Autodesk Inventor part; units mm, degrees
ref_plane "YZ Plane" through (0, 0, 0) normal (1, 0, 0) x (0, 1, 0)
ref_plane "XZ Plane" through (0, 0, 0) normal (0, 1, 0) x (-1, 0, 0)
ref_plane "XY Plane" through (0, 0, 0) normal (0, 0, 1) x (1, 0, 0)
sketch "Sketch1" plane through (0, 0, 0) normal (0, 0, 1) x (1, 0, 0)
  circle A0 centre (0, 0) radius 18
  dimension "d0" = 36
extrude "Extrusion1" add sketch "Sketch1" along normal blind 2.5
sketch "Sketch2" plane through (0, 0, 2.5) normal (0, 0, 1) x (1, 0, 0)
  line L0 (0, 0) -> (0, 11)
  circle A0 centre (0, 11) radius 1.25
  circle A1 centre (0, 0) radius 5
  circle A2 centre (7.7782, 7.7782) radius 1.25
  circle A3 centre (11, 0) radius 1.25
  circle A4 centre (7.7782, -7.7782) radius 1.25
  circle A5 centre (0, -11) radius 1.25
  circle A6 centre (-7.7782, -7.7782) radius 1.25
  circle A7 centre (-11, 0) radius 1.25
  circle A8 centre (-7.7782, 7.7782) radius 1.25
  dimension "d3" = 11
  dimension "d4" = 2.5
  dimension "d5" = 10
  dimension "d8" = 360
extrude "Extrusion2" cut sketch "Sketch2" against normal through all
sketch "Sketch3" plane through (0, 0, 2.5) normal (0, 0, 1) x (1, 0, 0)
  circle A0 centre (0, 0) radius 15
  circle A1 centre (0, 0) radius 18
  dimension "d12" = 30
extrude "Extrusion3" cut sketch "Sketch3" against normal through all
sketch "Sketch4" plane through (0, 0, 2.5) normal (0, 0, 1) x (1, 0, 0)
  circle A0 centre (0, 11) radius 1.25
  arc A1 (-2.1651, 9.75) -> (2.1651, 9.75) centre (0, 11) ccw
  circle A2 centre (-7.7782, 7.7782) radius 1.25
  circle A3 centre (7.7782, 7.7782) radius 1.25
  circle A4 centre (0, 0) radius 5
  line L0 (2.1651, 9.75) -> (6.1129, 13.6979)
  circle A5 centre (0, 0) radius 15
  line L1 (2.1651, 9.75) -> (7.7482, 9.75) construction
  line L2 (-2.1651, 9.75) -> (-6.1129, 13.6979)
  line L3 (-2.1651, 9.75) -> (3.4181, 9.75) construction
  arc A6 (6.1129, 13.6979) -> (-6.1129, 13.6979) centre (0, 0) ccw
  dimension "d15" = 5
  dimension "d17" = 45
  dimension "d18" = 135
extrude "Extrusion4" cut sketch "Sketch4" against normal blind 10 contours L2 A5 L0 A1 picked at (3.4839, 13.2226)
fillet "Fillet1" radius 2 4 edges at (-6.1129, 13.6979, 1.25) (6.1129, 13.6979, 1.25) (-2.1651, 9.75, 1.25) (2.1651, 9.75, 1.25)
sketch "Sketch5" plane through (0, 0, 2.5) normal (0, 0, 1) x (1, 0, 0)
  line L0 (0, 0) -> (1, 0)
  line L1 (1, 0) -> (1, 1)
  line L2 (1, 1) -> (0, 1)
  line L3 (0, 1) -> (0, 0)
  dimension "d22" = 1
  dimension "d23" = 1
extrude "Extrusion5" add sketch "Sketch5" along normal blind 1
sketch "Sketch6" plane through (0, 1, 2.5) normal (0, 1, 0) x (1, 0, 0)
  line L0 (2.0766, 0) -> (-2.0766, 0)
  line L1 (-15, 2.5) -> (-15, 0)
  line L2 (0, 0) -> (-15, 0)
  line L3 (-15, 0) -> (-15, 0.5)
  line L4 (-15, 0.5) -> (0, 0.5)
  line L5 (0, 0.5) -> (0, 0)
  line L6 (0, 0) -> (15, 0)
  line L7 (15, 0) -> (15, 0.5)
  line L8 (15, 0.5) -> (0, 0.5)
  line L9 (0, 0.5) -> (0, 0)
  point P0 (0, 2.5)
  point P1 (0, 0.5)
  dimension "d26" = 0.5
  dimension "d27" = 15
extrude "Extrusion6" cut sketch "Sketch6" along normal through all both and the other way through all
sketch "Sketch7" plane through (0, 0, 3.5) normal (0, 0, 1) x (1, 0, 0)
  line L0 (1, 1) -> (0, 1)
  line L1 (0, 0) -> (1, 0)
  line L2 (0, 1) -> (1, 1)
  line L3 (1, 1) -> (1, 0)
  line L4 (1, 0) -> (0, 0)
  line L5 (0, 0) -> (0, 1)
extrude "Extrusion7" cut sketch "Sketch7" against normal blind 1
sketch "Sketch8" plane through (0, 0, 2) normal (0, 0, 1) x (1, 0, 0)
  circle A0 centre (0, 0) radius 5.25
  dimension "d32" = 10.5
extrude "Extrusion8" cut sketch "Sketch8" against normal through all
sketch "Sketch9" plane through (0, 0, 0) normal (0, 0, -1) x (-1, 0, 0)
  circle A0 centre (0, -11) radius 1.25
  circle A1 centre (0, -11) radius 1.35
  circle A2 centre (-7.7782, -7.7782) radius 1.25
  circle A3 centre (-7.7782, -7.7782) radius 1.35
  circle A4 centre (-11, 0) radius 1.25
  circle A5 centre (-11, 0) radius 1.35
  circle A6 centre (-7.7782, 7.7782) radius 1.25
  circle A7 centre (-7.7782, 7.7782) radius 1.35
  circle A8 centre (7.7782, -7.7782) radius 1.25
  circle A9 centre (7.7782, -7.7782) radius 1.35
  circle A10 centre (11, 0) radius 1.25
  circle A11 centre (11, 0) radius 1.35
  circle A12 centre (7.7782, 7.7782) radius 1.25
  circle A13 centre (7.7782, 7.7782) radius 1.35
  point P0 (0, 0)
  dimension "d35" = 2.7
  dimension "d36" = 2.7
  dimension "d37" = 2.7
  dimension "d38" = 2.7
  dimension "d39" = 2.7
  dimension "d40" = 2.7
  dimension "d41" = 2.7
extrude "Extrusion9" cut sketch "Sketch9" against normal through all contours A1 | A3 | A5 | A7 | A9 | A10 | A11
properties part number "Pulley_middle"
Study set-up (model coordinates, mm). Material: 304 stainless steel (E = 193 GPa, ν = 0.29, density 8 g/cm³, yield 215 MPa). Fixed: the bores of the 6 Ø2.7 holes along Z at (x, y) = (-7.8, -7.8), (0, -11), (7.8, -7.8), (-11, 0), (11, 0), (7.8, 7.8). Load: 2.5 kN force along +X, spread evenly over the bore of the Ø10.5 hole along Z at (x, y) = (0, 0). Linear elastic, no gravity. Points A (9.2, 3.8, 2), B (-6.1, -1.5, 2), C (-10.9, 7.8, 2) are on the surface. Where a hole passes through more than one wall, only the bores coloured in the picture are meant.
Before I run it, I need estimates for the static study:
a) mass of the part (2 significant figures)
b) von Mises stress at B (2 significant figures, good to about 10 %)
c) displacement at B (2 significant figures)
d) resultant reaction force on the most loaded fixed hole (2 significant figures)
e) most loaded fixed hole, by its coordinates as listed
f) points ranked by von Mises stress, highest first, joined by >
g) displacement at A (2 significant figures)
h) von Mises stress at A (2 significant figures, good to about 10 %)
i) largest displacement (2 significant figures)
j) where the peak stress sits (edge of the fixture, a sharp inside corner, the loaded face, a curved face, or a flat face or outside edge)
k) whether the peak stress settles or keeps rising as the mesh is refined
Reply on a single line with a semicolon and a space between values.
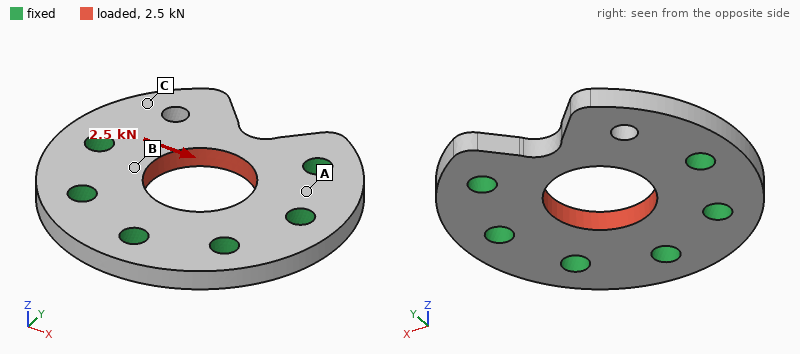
8.5 g; 46 MPa; 0.91 µm; 670 N; (-11, 0); B > A > C; 0.53 µm; 20 MPa; 2.8 µm; edge of the fixture; keeps rising
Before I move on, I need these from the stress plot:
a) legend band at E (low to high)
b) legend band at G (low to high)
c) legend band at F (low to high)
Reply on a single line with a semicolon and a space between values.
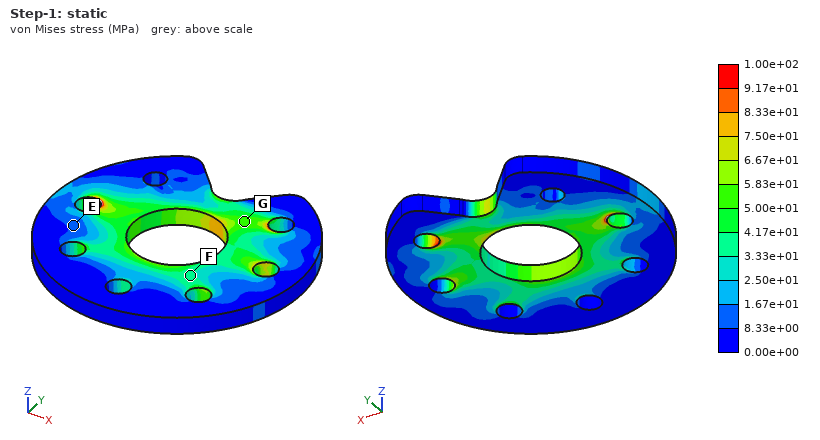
8.33e+00 to 1.67e+01 MPa; 5.00e+01 to 5.83e+01 MPa; 3.33e+01 to 4.17e+01 MPa
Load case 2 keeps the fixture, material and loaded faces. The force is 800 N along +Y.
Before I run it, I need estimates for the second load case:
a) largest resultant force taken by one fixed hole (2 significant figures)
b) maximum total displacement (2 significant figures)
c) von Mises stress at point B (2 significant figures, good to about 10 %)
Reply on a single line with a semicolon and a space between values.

180 N; 1.8 µm; 22 MPa
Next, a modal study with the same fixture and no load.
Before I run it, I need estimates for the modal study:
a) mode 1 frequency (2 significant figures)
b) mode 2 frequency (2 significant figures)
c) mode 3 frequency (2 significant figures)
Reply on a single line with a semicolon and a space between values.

15 kHz; 35 kHz; 49 kHz
